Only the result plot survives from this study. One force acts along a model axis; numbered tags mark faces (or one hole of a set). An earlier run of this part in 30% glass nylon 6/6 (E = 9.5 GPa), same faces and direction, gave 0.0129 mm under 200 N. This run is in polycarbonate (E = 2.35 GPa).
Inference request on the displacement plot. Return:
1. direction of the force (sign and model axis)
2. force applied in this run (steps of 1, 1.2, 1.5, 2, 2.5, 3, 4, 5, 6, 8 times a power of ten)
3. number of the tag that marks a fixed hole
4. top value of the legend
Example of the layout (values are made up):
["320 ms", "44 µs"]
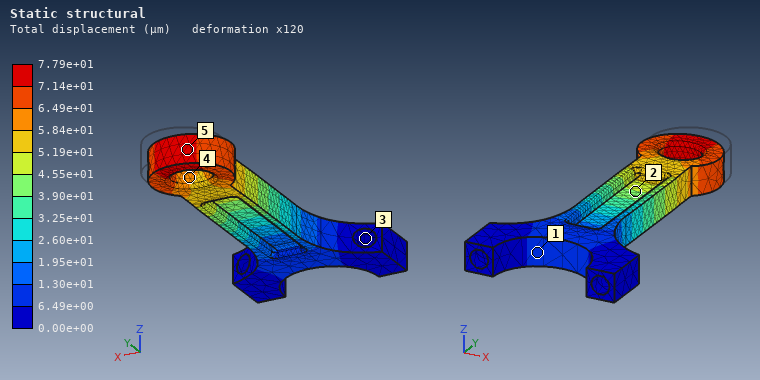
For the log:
["-Y", "300 N", "3", "7.79e+01 µm"]
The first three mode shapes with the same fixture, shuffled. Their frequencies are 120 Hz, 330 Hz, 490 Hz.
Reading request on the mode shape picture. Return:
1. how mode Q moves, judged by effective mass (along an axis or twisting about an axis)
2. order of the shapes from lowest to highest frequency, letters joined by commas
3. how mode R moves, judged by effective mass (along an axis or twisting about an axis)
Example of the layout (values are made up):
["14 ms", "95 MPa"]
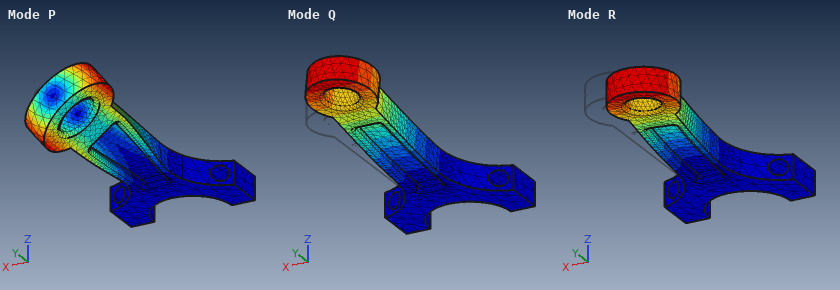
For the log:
["along Z", "Q, R, P", "along X"]
